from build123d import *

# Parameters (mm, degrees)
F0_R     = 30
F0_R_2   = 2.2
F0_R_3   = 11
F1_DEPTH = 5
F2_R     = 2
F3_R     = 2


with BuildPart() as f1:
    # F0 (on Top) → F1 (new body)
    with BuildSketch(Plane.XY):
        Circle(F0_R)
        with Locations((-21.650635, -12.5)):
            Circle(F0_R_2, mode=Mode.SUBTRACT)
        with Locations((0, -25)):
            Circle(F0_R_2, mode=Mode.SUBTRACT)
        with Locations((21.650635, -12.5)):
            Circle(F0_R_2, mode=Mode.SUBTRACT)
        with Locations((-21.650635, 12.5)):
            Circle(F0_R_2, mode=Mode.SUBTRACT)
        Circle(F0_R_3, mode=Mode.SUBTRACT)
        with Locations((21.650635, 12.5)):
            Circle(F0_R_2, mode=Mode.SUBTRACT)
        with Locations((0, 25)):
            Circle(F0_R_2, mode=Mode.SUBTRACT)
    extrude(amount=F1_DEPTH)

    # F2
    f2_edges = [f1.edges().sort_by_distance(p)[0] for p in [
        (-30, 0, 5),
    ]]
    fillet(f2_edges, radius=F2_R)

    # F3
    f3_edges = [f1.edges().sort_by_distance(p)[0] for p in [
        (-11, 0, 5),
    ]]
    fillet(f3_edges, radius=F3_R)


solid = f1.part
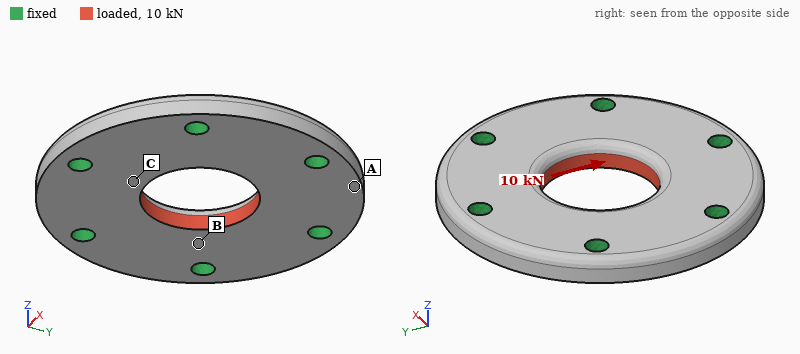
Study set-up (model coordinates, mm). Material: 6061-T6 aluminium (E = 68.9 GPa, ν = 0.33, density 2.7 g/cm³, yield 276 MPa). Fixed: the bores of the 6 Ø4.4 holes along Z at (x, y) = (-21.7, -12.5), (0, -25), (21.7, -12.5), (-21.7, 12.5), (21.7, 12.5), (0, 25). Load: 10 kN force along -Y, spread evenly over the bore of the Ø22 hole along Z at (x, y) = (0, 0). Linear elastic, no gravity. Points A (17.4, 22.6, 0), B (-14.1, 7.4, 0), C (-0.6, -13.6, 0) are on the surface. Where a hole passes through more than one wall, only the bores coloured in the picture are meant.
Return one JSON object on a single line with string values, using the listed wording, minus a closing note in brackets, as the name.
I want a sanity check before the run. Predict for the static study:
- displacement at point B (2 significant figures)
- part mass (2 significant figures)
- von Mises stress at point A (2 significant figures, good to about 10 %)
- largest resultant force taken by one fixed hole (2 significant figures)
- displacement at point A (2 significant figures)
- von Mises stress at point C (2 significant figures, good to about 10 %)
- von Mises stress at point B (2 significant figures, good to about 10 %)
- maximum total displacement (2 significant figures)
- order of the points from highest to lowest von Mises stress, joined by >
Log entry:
{"displacement at point B": "4.4 µm", "part mass": "31 g", "von Mises stress at point A": "11 MPa", "largest resultant force taken by one fixed hole": "2.4 kN", "displacement at point A": "3.7 µm", "von Mises stress at point C": "58 MPa", "von Mises stress at point B": "30 MPa", "maximum total displacement": "11 µm", "order of the points from highest to lowest von Mises stress, joined by >": "C > B > A"}
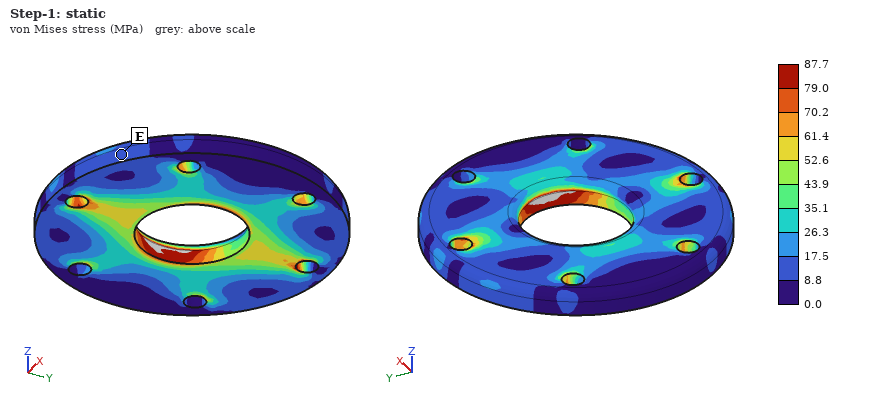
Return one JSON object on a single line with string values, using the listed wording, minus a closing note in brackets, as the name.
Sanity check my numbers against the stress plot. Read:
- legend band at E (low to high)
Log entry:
{"legend band at E": "8.8 to 17.5 MPa"}
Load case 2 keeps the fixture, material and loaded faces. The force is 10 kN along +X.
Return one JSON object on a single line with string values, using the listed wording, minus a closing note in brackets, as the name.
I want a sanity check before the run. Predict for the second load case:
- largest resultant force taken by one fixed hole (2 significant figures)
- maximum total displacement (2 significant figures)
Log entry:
{"largest resultant force taken by one fixed hole": "2.1 kN", "maximum total displacement": "12 µm"}
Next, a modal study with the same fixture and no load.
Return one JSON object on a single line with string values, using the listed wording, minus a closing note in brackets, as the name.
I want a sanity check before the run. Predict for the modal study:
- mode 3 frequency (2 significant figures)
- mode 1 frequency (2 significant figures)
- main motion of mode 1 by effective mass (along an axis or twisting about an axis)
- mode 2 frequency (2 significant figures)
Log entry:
{"mode 3 frequency": "29 kHz", "mode 1 frequency": "22 kHz", "main motion of mode 1 by effective mass": "along Z", "mode 2 frequency": "29 kHz"}
